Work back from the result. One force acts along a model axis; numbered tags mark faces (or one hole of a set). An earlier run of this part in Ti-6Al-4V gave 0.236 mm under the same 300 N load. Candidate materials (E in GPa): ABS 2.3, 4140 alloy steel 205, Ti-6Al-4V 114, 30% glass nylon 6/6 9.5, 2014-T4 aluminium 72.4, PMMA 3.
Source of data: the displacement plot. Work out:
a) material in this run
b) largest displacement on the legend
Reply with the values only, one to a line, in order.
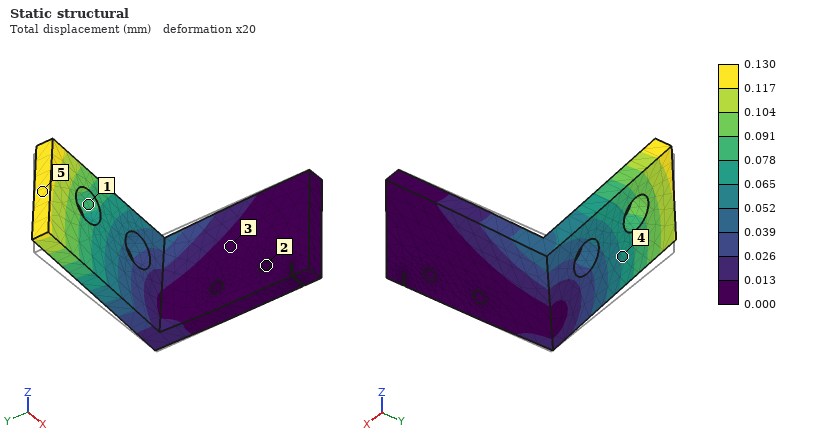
4140 alloy steel
0.130 mm
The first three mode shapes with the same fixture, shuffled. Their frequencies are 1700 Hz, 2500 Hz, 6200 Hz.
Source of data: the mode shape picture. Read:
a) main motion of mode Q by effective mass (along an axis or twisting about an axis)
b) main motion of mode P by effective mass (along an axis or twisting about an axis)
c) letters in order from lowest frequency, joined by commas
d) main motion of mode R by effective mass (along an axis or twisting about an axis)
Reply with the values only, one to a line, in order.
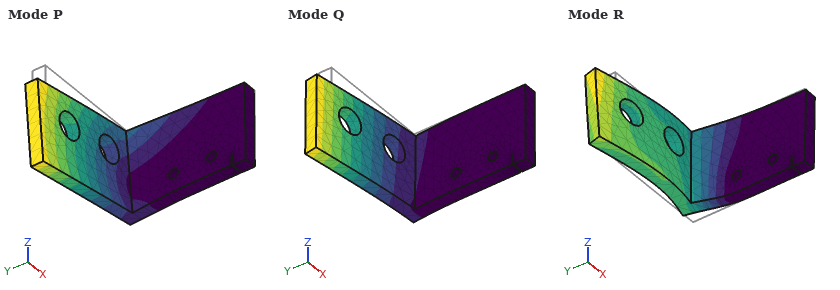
along Y
along Z
Q, P, R
along X
